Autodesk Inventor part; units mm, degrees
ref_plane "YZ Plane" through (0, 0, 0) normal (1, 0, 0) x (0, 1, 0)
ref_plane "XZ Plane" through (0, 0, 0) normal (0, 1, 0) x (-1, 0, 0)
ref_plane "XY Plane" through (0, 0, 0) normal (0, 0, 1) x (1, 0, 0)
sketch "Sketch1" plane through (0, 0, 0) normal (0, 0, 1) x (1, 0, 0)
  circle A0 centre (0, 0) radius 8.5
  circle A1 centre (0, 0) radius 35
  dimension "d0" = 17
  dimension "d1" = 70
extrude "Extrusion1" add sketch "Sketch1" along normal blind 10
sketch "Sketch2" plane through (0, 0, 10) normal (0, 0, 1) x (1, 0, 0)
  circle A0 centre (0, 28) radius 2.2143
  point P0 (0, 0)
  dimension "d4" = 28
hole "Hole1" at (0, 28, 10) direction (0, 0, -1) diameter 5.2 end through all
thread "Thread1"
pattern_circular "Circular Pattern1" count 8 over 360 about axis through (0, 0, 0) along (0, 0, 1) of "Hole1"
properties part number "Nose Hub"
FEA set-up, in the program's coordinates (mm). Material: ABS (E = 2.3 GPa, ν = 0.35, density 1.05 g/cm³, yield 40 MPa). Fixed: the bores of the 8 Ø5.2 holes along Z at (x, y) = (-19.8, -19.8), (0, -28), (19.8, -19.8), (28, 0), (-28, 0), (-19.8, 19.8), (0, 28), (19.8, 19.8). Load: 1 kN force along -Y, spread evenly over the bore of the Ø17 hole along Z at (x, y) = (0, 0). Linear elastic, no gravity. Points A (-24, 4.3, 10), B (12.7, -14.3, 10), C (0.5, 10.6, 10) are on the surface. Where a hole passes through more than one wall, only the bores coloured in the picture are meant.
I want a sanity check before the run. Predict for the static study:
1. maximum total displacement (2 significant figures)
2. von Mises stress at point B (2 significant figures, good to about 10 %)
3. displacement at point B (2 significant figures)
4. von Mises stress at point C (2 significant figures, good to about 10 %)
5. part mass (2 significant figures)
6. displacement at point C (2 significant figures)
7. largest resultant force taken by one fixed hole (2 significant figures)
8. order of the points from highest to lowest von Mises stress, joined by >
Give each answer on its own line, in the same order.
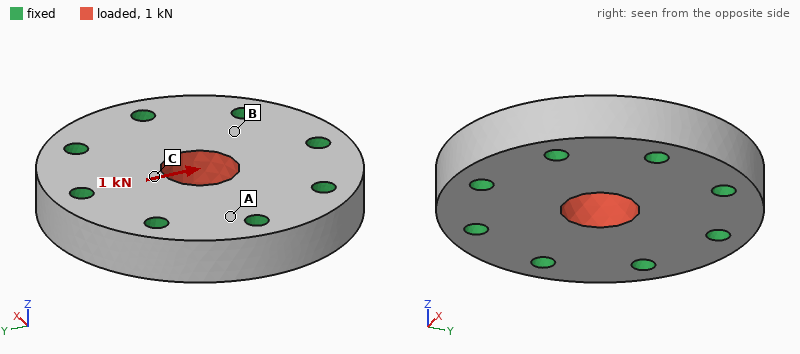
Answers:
14 µm
1.2 MPa
4.7 µm
1.9 MPa
36 g
12 µm
210 N
C > B > A
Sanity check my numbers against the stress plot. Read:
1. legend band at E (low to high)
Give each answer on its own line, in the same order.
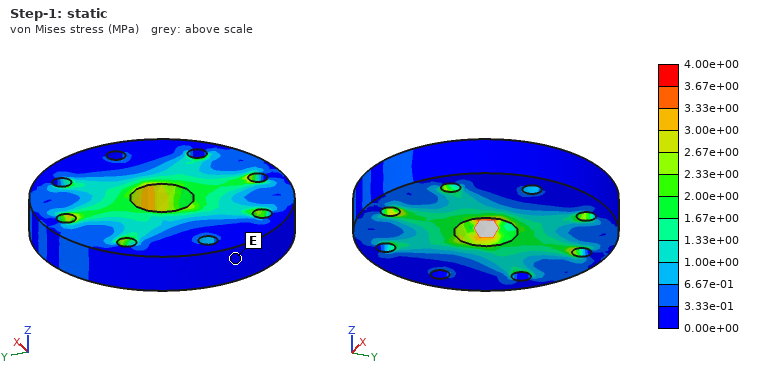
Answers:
0.00e+00 to 3.33e-01 MPa
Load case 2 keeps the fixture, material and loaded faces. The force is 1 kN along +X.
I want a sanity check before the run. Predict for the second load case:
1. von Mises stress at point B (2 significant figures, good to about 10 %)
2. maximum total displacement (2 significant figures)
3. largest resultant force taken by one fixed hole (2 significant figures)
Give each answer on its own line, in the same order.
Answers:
1.2 MPa
14 µm
210 N
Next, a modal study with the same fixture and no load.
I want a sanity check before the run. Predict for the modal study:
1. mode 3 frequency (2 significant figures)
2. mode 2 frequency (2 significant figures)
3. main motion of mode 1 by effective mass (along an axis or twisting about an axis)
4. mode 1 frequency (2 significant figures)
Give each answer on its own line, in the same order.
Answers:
11 kHz
11 kHz
along Z
7600 Hz
